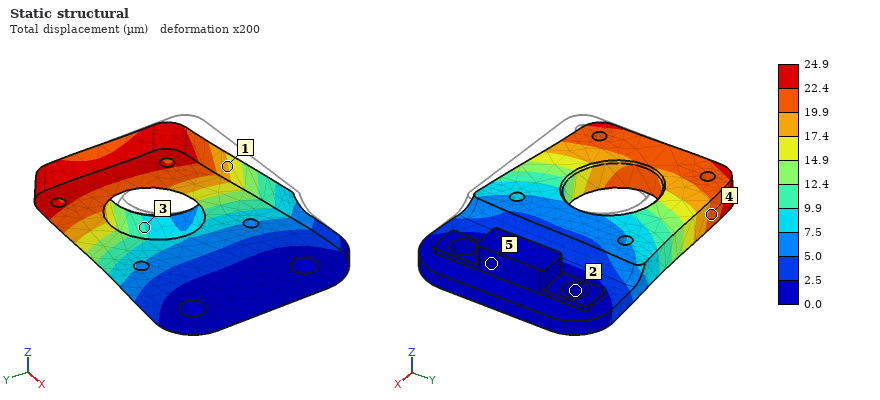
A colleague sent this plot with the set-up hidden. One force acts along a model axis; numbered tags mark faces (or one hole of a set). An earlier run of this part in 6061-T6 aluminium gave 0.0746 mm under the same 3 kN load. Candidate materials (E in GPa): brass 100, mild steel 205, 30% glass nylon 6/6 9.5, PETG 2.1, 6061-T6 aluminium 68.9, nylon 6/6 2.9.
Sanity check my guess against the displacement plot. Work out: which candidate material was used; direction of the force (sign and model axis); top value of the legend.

mild steel
+Y
24.9 µm
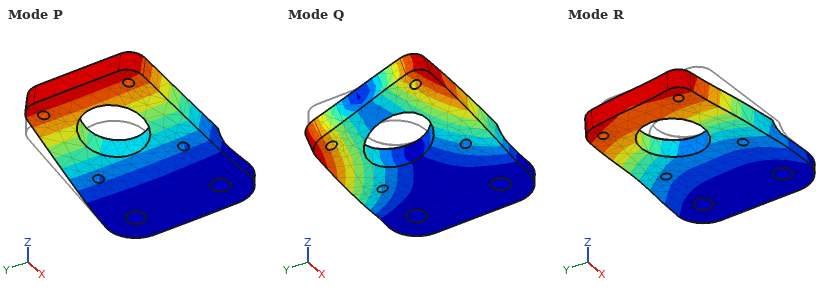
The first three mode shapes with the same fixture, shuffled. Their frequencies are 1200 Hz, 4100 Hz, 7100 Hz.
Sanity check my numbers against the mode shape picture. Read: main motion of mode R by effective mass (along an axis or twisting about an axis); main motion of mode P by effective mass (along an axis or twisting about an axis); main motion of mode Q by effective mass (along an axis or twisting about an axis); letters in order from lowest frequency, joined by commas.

along Y
along Z
twisting about X
P, Q, R
